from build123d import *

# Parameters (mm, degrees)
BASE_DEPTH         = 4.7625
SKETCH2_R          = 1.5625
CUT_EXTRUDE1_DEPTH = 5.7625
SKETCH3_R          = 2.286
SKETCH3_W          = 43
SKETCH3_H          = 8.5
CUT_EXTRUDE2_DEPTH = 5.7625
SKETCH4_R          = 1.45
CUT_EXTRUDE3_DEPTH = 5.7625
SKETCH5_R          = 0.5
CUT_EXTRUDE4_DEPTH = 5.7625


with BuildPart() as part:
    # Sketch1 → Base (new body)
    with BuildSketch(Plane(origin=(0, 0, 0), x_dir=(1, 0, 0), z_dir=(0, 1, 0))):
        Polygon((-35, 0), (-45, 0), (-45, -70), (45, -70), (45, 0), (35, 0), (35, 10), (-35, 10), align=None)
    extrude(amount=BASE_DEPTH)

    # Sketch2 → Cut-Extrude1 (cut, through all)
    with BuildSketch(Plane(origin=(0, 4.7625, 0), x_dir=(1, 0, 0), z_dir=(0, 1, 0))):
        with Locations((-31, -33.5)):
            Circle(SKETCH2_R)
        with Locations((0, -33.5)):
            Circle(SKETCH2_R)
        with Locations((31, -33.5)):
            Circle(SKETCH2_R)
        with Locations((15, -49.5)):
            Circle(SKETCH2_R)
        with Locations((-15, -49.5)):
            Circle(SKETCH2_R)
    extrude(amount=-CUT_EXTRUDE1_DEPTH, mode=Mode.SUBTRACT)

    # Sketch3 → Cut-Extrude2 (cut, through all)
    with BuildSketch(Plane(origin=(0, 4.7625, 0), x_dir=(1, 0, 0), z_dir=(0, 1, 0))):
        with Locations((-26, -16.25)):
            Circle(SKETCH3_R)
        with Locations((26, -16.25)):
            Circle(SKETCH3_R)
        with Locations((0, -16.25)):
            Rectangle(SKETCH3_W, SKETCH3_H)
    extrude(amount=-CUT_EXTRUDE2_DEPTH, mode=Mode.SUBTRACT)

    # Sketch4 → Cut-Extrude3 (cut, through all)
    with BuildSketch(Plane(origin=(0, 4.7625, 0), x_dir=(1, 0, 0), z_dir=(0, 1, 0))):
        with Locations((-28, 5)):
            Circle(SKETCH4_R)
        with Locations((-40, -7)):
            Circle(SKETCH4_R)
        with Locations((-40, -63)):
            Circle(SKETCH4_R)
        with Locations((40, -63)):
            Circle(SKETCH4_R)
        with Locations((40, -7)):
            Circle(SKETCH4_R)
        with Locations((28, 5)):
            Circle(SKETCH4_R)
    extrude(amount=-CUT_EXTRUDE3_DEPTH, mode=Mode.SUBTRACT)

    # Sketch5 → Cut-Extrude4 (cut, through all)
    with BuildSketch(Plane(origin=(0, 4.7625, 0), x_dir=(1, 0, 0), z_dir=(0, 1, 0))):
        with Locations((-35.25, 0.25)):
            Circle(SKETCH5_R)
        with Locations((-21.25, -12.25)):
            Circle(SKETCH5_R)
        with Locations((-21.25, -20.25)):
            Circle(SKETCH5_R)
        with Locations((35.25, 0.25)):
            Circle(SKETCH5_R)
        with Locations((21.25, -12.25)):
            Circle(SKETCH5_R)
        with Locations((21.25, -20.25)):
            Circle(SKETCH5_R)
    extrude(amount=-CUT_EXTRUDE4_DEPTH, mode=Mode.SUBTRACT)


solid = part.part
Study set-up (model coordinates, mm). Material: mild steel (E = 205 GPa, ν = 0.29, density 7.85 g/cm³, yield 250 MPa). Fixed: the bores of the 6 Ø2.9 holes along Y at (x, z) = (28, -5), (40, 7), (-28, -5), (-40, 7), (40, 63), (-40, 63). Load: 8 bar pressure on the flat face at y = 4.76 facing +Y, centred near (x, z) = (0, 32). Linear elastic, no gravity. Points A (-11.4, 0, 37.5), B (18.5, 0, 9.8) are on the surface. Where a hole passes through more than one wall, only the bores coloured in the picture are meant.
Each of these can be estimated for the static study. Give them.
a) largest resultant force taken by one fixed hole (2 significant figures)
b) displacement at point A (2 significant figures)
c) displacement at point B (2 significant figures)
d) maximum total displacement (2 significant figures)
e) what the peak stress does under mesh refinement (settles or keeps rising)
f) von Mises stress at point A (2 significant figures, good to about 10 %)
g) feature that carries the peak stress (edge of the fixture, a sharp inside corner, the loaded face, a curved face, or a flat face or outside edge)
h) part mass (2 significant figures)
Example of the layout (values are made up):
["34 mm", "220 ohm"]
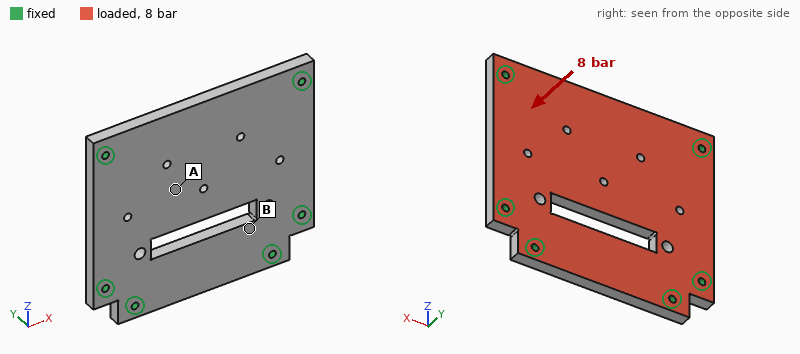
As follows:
["1.2 kN", "72 µm", "27 µm", "80 µm", "keeps rising", "46 MPa", "edge of the fixture", "240 g"]
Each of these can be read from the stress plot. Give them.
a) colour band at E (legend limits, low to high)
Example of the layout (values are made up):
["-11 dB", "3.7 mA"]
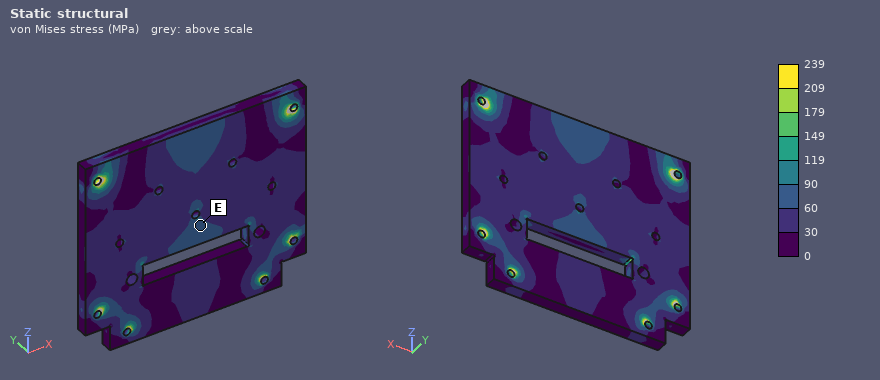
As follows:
["60 to 90 MPa"]
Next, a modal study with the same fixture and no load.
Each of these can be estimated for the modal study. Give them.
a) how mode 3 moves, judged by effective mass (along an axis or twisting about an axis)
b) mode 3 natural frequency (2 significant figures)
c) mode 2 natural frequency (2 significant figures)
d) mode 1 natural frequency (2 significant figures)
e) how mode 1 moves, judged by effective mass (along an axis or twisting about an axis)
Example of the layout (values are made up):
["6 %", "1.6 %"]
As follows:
["twisting about Z", "6700 Hz", "5300 Hz", "3100 Hz", "along Y"]
